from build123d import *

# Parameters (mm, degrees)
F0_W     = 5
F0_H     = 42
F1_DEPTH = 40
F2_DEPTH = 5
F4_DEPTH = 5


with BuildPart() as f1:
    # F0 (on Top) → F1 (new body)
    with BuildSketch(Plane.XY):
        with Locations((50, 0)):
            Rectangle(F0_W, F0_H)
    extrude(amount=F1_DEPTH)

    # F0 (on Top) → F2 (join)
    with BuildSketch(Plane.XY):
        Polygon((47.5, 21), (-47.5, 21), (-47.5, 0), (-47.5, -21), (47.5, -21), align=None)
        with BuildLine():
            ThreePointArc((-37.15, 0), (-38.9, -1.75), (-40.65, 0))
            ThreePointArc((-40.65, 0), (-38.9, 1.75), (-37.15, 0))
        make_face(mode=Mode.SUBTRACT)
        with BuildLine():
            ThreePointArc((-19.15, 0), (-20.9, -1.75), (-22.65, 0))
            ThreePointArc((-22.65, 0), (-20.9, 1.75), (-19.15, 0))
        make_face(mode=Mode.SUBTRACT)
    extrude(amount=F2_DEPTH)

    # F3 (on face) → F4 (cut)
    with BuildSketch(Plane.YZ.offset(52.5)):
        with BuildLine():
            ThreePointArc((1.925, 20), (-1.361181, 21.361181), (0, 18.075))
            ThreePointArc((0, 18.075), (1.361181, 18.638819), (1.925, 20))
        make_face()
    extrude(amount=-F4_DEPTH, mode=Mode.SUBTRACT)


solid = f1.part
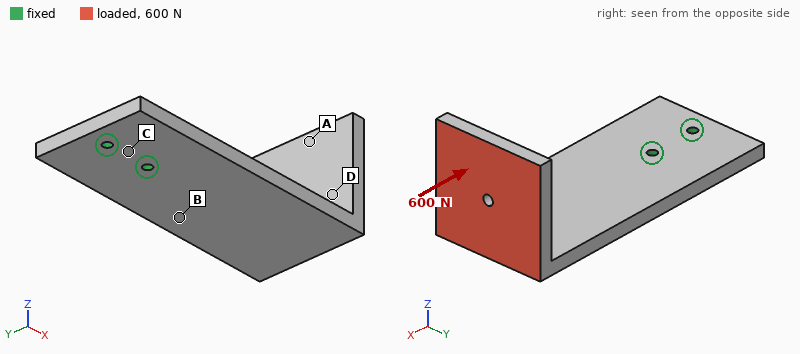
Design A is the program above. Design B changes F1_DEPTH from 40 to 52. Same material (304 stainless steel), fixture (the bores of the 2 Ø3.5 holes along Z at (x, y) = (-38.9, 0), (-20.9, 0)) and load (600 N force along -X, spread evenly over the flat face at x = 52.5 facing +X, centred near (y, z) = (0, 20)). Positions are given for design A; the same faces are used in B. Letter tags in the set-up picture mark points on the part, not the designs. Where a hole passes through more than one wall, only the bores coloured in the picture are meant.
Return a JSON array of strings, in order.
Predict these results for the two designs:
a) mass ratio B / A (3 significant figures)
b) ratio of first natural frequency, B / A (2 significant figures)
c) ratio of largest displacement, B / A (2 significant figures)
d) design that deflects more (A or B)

["1.09", "0.86", "1.6", "B"]
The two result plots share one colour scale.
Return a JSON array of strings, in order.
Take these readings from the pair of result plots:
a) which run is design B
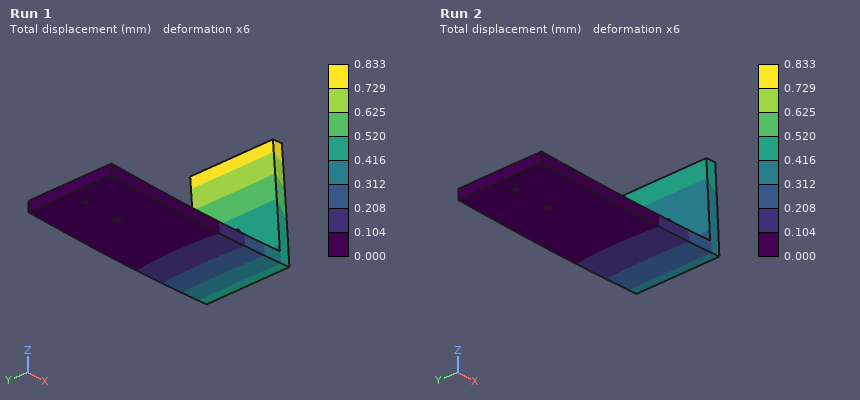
["Run 1"]
